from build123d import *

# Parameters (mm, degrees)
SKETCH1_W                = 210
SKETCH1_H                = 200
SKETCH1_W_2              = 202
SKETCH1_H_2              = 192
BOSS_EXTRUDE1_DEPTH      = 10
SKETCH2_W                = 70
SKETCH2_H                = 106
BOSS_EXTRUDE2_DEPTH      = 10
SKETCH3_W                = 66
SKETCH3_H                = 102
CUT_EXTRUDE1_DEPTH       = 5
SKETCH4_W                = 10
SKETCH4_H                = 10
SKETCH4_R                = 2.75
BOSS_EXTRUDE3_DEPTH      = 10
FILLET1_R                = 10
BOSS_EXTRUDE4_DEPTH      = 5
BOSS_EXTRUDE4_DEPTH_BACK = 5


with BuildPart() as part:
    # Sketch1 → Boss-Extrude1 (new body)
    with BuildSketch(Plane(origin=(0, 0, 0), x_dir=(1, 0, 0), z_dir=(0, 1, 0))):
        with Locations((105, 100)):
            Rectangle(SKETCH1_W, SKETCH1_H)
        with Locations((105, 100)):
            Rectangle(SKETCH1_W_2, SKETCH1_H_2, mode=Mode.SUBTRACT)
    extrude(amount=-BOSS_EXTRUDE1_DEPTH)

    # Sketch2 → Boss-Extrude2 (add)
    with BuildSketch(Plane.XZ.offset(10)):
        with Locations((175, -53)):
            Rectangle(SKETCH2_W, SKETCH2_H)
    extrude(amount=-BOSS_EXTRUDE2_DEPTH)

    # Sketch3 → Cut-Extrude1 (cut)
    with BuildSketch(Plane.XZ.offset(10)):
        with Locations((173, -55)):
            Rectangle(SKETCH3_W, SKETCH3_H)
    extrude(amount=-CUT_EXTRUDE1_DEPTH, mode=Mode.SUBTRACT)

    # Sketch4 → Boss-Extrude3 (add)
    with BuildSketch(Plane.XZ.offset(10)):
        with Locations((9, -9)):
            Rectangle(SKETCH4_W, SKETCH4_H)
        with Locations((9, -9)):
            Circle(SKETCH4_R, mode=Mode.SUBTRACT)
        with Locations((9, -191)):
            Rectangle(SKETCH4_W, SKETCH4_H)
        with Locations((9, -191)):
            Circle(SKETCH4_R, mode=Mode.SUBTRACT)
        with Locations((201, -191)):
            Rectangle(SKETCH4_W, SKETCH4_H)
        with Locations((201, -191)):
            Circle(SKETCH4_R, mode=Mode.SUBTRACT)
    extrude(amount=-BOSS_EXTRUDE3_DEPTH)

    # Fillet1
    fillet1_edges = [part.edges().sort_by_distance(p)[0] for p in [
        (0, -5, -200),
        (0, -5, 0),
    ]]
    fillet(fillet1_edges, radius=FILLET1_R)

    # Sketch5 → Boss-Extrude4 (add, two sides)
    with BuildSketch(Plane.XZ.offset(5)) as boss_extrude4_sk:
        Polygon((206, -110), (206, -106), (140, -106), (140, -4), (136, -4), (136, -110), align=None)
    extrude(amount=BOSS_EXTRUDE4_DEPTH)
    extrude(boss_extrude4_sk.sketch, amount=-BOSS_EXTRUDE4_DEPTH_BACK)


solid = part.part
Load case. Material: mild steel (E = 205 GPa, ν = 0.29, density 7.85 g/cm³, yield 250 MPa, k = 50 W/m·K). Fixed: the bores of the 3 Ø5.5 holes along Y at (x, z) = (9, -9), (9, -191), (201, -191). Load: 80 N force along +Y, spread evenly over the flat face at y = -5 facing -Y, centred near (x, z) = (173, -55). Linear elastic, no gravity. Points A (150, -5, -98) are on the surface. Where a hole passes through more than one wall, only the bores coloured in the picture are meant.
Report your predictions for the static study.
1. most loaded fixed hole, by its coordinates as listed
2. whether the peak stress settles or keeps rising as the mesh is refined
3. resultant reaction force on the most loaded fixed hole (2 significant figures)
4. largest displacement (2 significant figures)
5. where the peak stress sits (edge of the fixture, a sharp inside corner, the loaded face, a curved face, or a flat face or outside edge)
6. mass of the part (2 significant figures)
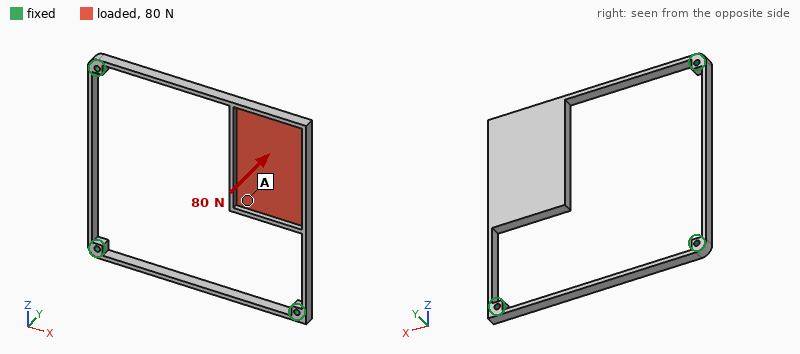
(201, -191)
keeps rising
46 N
0.46 mm
a sharp inside corner
590 g
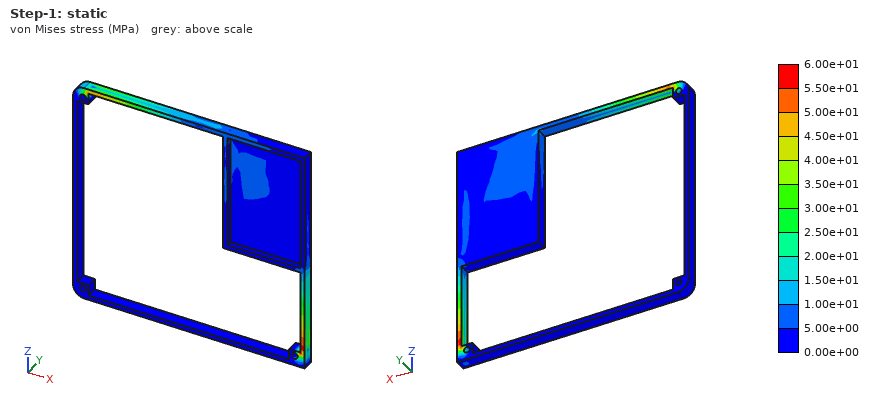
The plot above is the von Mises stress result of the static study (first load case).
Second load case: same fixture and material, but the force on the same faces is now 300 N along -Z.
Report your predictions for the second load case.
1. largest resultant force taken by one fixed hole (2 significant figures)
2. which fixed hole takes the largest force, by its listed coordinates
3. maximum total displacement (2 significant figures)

290 N
(201, -191)
0.21 mm
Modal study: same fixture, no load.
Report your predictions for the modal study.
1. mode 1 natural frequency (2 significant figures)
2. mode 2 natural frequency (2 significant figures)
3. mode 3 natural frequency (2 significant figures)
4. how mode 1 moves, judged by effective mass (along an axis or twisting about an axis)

140 Hz
270 Hz
380 Hz
along Y
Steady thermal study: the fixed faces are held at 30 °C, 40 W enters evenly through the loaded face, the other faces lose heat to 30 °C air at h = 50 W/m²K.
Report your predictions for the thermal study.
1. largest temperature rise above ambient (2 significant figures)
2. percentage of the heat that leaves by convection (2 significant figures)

55 K
98 %
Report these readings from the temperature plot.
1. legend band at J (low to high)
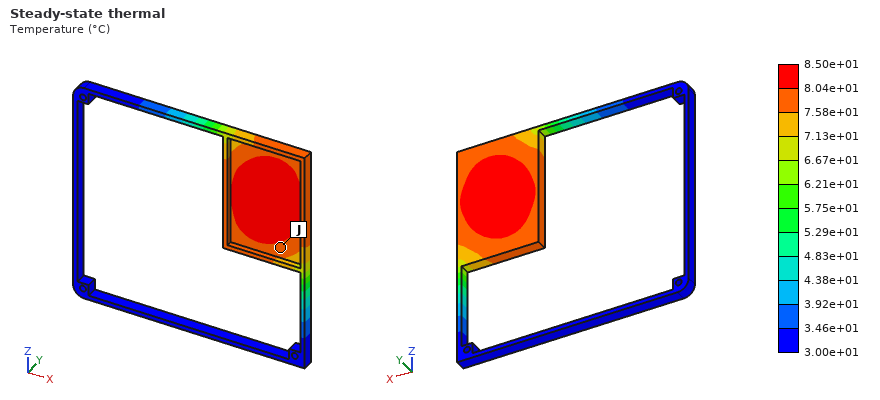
7.58e+01 to 8.04e+01 °C
